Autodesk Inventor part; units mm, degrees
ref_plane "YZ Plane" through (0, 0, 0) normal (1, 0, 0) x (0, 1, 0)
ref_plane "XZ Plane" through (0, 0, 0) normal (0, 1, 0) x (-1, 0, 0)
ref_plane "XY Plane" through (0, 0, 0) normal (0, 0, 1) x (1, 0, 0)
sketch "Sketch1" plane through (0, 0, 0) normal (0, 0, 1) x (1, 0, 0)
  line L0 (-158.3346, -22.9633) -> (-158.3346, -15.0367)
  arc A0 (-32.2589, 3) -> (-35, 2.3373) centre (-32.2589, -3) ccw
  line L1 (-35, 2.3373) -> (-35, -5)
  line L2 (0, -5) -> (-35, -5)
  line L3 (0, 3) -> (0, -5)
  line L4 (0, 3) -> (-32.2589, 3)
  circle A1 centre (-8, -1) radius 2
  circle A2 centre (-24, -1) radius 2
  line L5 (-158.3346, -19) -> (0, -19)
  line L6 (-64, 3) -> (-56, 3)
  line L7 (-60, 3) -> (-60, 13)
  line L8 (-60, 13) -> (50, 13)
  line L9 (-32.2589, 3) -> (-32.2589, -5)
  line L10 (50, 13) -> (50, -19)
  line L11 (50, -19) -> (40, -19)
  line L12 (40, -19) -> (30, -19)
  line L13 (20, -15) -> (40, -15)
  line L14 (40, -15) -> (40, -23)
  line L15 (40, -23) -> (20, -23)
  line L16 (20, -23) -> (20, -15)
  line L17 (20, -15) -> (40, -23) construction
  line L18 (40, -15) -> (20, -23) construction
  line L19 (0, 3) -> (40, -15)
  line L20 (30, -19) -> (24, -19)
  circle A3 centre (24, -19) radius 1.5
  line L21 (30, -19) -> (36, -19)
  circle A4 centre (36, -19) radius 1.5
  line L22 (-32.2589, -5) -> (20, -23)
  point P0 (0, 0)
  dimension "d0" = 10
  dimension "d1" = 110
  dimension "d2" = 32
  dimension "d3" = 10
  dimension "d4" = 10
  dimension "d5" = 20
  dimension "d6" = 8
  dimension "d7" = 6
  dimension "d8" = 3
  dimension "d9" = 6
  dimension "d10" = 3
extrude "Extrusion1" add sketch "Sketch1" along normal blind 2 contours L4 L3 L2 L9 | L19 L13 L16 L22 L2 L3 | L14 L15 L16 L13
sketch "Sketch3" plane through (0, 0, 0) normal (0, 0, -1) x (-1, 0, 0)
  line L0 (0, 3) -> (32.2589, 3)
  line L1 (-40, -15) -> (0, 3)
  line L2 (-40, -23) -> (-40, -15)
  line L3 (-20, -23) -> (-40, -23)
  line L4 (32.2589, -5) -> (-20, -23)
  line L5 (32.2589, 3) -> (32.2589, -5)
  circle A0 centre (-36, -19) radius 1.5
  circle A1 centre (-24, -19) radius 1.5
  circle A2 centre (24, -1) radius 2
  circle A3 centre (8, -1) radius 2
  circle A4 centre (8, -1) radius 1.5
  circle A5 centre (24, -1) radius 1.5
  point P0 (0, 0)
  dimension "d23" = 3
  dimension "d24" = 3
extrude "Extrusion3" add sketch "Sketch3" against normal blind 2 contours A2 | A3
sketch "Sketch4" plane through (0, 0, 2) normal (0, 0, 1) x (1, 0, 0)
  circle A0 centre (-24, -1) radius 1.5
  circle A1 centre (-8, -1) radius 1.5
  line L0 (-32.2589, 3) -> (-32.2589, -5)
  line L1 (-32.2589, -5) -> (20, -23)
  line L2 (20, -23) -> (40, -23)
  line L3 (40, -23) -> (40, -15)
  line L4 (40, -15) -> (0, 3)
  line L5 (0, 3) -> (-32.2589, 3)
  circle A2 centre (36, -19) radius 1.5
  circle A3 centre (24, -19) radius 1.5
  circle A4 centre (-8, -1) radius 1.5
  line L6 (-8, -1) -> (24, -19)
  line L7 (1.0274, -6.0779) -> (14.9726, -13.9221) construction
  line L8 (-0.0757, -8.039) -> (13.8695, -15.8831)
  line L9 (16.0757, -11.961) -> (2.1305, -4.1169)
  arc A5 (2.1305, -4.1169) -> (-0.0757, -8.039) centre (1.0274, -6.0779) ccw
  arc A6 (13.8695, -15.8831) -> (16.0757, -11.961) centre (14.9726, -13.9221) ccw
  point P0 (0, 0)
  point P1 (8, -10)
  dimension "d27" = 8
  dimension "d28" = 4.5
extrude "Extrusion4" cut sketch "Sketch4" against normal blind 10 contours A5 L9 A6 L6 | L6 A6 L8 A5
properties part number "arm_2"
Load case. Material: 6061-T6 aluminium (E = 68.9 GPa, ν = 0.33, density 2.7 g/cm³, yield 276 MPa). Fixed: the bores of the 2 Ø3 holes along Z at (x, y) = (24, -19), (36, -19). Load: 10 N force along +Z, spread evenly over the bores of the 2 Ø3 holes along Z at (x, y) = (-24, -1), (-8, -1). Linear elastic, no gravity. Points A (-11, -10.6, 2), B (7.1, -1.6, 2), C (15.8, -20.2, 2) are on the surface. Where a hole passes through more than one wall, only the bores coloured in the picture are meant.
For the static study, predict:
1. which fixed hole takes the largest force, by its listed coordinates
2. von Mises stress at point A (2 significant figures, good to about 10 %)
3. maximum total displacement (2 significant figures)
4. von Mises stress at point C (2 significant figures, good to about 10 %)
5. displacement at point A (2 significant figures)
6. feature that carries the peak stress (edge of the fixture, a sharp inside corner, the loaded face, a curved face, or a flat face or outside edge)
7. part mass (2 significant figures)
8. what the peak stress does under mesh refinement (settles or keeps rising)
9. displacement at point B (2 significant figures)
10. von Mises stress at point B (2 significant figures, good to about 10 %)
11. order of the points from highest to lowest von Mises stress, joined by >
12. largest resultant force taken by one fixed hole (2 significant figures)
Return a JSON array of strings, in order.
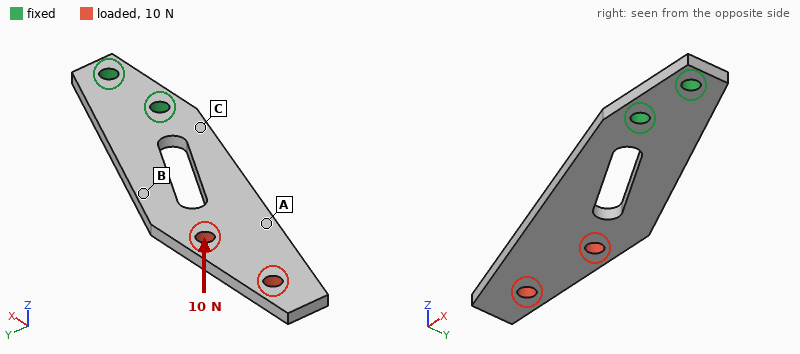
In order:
["(24, -19)", "9.0 MPa", "0.71 mm", "43 MPa", "0.32 mm", "edge of the fixture", "5.0 g", "keeps rising", "0.14 mm", "27 MPa", "C > B > A", "22 N"]
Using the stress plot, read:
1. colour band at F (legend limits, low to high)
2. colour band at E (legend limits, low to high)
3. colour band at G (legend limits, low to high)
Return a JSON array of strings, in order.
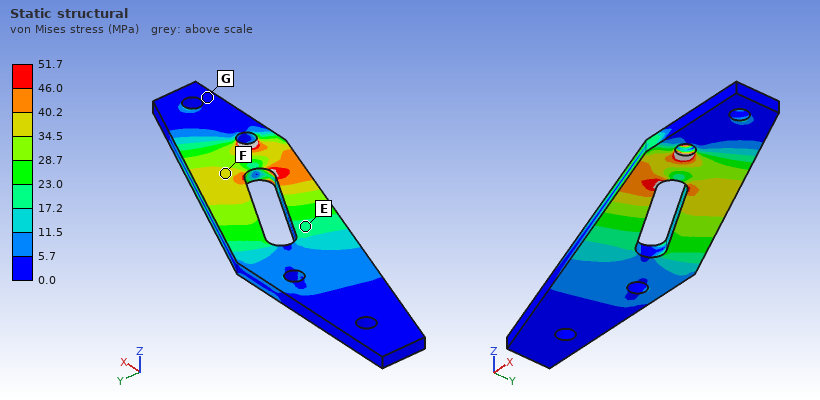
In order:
["34.5 to 40.2 MPa", "17.2 to 23.0 MPa", "0.0 to 5.7 MPa"]
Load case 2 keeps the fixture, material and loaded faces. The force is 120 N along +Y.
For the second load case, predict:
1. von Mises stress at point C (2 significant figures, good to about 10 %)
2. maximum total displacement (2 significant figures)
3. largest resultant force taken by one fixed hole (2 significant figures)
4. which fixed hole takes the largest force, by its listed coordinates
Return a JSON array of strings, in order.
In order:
["51 MPa", "0.19 mm", "450 N", "(24, -19)"]
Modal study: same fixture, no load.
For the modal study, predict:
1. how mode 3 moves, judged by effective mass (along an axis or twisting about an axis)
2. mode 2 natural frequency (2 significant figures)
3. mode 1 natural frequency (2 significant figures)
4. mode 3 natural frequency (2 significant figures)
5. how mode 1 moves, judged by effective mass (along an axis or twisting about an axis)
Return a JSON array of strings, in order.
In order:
["along Y", "2800 Hz", "510 Hz", "3000 Hz", "along Z"]
